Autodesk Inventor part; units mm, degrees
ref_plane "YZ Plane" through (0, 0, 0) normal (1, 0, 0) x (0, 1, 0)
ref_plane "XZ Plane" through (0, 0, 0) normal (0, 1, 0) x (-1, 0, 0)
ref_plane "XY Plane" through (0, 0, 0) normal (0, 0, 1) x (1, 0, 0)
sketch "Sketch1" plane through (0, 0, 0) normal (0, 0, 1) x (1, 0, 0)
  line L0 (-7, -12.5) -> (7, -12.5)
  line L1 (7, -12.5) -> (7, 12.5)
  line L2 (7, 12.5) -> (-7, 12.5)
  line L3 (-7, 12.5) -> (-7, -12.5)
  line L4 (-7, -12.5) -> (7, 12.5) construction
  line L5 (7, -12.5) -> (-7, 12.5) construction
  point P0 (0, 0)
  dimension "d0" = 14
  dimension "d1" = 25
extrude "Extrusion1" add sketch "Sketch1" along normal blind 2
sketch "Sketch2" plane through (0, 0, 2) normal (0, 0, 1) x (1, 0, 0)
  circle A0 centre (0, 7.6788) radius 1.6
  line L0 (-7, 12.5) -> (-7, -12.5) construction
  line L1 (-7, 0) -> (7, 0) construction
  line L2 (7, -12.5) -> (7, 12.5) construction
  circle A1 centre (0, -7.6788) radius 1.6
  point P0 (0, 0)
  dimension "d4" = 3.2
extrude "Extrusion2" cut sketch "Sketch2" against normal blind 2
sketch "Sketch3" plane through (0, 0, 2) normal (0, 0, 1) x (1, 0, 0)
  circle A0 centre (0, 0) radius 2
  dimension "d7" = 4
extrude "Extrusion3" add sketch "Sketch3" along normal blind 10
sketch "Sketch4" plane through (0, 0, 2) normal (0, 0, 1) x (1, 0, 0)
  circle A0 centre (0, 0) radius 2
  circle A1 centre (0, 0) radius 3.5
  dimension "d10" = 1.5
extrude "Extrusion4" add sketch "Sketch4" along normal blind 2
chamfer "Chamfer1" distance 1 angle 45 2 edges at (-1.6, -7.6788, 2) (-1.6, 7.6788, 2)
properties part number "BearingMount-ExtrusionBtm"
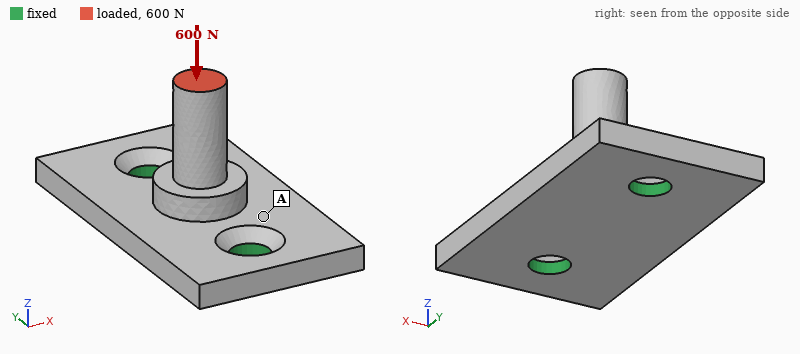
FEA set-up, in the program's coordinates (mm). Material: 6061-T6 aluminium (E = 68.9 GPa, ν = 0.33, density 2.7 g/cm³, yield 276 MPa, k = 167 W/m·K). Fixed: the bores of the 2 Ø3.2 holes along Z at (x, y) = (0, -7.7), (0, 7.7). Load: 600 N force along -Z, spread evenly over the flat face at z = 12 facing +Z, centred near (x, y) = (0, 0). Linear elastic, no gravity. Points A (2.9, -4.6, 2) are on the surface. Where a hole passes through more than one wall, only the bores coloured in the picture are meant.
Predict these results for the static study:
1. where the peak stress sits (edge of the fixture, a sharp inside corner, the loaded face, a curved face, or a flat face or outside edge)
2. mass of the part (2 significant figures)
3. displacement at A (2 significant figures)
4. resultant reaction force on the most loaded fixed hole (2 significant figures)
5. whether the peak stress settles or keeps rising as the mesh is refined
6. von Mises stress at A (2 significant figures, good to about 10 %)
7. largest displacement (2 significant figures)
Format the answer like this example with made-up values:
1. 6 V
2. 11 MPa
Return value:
1. edge of the fixture
2. 2.2 g
3. 8.2 µm
4. 390 N
5. keeps rising
6. 32 MPa
7. 20 µm
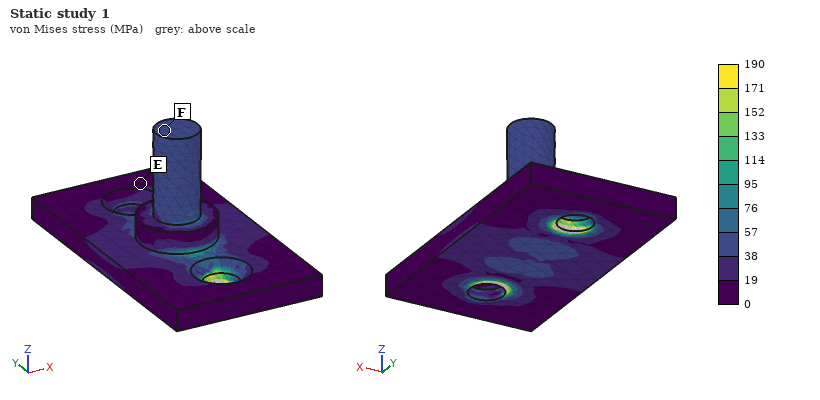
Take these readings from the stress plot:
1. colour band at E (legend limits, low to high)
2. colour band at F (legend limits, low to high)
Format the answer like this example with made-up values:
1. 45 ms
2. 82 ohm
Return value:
1. 0 to 19 MPa
2. 38 to 57 MPa
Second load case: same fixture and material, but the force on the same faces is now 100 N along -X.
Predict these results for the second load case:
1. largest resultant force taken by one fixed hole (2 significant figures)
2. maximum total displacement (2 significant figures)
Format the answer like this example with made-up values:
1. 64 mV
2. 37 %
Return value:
1. 50 N
2. 73 µm
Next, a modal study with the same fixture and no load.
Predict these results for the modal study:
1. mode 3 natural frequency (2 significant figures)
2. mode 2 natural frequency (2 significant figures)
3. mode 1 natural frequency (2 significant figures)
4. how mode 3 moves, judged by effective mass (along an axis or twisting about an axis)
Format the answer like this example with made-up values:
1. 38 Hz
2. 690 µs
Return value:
1. 29 kHz
2. 27 kHz
3. 15 kHz
4. along Z
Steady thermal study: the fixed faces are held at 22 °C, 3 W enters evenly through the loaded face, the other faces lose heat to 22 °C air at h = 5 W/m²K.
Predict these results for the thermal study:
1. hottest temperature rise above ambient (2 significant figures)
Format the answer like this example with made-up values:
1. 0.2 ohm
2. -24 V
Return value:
1. 16 K
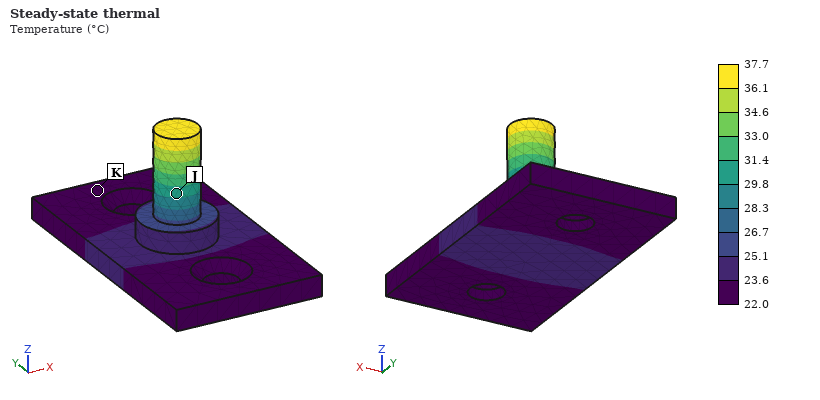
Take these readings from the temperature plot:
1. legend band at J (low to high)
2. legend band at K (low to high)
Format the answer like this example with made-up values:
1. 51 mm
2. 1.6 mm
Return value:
1. 29.8 to 31.4 °C
2. 22.0 to 23.6 °C
